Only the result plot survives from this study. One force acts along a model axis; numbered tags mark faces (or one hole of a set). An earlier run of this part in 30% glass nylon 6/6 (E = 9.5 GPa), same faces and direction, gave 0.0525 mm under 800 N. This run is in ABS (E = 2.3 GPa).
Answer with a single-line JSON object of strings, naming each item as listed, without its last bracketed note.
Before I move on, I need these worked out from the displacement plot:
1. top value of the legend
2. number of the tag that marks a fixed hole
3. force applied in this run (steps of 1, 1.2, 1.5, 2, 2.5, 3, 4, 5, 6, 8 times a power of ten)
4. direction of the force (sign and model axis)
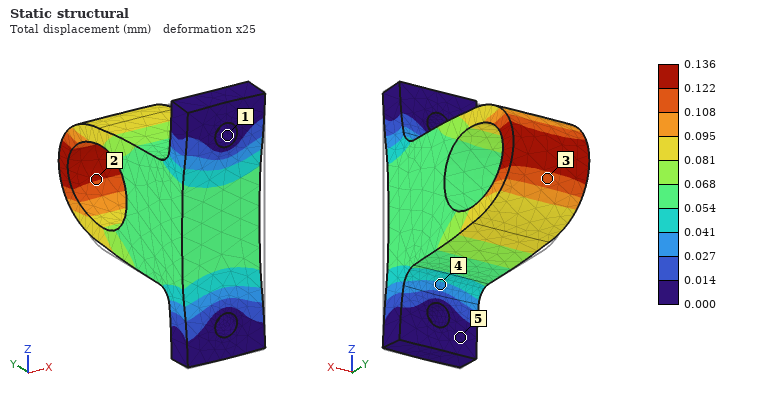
{"top value of the legend": "0.136 mm", "number of the tag that marks a fixed hole": "1", "force applied in this run": "500 N", "direction of the force": "+Y"}
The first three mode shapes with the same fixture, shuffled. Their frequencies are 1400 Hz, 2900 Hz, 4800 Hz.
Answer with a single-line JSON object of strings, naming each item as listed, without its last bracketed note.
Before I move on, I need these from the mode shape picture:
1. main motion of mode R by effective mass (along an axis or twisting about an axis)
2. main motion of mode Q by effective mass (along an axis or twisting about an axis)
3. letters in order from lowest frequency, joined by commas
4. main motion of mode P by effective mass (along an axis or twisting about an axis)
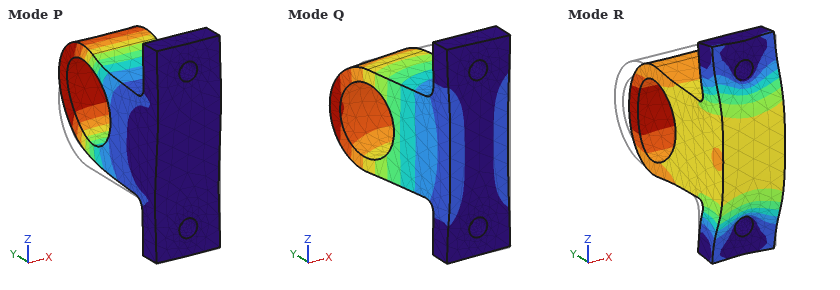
{"main motion of mode R by effective mass": "along Y", "main motion of mode Q by effective mass": "along X", "letters in order from lowest frequency, joined by commas": "Q, P, R", "main motion of mode P by effective mass": "along Z"}
